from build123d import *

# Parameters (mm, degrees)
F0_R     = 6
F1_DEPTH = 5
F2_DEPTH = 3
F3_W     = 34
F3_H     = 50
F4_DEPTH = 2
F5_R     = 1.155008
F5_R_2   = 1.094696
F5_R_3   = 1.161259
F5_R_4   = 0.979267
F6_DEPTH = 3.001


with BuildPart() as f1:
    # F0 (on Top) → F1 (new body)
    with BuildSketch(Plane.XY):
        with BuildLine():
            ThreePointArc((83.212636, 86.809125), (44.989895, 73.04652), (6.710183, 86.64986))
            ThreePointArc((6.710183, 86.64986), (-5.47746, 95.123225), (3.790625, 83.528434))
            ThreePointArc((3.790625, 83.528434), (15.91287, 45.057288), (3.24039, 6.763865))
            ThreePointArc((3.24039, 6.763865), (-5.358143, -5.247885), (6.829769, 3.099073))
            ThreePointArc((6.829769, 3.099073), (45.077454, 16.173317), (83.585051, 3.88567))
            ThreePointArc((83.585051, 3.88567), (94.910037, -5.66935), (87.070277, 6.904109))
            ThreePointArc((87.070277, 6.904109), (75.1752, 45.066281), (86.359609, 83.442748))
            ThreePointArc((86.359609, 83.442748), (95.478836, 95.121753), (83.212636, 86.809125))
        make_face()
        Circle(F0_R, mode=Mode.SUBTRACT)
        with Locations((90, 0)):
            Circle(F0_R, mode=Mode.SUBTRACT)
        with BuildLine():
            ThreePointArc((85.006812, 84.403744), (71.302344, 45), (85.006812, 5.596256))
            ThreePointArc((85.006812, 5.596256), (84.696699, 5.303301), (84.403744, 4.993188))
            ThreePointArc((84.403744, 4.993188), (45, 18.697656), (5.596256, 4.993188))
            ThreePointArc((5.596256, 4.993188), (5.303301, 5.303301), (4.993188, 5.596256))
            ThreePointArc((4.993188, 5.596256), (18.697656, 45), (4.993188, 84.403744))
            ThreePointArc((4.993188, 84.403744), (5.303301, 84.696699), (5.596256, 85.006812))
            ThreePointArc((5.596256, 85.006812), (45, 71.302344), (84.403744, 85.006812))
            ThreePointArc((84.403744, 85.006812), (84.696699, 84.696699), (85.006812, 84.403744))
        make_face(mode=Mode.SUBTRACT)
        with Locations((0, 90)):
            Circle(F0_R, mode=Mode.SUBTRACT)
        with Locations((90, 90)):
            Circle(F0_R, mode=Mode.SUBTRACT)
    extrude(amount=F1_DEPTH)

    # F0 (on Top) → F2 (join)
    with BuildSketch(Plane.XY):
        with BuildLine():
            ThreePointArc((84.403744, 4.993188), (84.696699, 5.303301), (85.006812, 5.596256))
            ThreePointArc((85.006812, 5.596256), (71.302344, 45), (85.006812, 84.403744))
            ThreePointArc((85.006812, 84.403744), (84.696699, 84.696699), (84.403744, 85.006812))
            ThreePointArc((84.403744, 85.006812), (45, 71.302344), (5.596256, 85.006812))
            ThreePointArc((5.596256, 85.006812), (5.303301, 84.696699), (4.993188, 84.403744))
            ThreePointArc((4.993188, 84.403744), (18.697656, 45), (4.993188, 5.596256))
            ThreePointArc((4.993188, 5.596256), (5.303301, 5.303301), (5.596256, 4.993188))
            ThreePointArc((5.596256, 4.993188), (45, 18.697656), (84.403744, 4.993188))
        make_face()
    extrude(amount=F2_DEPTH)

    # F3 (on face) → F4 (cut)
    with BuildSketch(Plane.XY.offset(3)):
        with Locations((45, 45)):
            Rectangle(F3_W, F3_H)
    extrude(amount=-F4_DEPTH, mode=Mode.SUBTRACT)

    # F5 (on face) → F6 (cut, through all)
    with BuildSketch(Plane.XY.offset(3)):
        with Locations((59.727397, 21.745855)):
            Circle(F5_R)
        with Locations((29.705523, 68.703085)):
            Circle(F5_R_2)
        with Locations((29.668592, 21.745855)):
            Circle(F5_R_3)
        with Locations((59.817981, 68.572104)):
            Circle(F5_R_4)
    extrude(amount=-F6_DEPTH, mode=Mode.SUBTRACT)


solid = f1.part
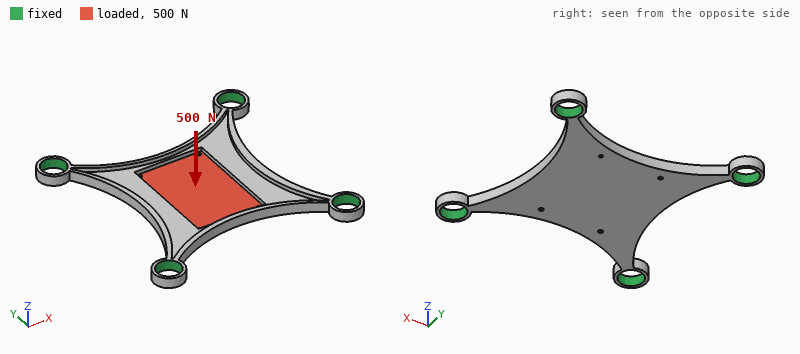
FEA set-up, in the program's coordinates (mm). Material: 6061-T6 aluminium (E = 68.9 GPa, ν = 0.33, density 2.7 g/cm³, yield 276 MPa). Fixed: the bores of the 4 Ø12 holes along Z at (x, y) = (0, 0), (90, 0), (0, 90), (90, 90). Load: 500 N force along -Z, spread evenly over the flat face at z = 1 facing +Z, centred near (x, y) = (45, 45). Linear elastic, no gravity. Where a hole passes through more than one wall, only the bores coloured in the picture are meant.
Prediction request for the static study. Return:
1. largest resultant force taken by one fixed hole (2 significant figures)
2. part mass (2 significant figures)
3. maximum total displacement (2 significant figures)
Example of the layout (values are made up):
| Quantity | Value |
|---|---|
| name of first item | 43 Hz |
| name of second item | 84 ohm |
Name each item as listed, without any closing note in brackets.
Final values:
| Quantity | Value |
|---|---|
| largest resultant force taken by one fixed hole | 600 N |
| part mass | 33 g |
| maximum total displacement | 0.50 mm |
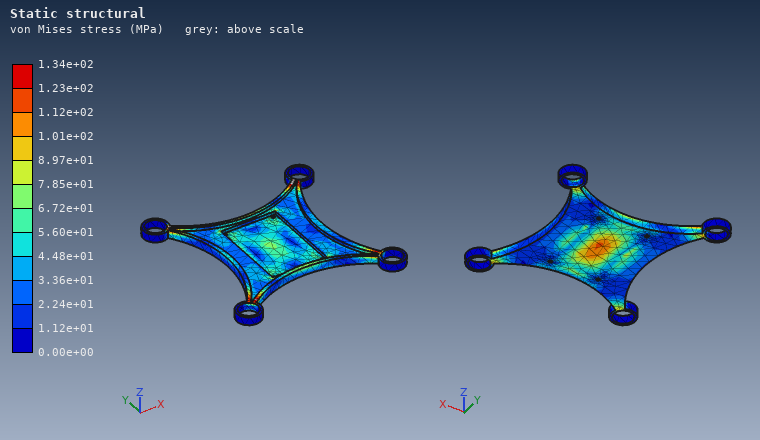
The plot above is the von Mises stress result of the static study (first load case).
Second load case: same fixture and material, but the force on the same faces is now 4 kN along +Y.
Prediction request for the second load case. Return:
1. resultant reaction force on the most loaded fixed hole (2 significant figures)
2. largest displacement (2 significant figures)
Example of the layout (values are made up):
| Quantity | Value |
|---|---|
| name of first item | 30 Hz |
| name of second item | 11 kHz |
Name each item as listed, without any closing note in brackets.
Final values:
| Quantity | Value |
|---|---|
| resultant reaction force on the most loaded fixed hole | 1.3 kN |
| largest displacement | 53 µm |
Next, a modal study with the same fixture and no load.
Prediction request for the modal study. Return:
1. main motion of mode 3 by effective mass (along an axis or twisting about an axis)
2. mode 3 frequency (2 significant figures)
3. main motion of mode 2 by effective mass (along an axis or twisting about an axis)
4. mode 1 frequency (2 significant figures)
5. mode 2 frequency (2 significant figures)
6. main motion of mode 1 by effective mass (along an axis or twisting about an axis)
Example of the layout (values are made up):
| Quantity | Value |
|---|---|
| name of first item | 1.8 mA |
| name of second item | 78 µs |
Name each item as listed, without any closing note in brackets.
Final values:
| Quantity | Value |
|---|---|
| main motion of mode 3 by effective mass | twisting about X |
| mode 3 frequency | 3500 Hz |
| main motion of mode 2 by effective mass | twisting about Y |
| mode 1 frequency | 1900 Hz |
| mode 2 frequency | 2800 Hz |
| main motion of mode 1 by effective mass | along Z |
